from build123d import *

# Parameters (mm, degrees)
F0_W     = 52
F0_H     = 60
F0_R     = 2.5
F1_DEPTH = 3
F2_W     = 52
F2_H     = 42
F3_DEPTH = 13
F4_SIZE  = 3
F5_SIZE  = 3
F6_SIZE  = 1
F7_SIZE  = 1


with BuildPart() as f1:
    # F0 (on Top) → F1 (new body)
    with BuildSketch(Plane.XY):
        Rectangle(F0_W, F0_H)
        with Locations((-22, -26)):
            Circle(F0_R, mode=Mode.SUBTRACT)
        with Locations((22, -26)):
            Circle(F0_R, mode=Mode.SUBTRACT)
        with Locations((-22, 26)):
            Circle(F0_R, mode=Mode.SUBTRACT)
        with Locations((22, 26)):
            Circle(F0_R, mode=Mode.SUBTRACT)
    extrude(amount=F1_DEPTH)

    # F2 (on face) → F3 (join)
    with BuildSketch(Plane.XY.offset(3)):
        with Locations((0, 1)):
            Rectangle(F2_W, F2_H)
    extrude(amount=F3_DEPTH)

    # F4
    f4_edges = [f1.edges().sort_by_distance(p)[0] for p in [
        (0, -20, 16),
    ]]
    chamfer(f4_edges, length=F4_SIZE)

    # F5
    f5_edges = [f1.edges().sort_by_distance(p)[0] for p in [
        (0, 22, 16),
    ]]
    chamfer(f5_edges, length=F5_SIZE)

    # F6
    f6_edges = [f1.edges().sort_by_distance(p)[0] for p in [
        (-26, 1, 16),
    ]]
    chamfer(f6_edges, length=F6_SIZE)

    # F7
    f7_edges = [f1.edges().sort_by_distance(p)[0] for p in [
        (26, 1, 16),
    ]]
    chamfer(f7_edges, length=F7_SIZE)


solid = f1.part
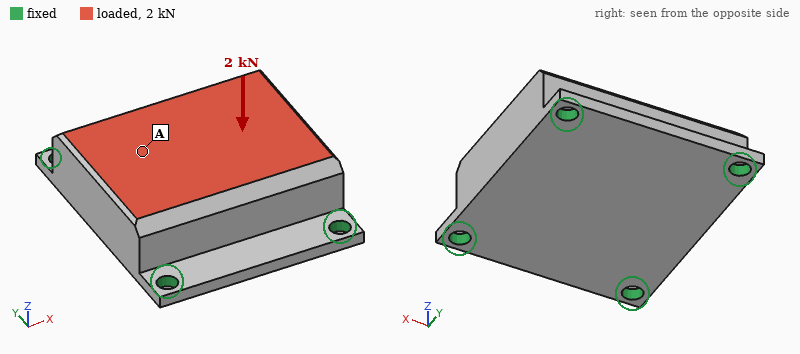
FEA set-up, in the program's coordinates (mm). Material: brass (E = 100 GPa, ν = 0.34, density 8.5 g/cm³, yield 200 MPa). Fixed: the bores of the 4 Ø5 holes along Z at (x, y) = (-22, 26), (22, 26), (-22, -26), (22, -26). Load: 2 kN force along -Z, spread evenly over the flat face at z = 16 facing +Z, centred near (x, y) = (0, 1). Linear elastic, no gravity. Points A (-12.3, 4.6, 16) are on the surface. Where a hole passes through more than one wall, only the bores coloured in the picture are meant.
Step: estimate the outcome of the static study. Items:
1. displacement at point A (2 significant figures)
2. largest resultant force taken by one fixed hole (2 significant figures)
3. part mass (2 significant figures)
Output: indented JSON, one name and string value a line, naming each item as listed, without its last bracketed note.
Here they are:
{
  "displacement at point A": "5.9 µm",
  "largest resultant force taken by one fixed hole": "620 N",
  "part mass": "310 g"
}
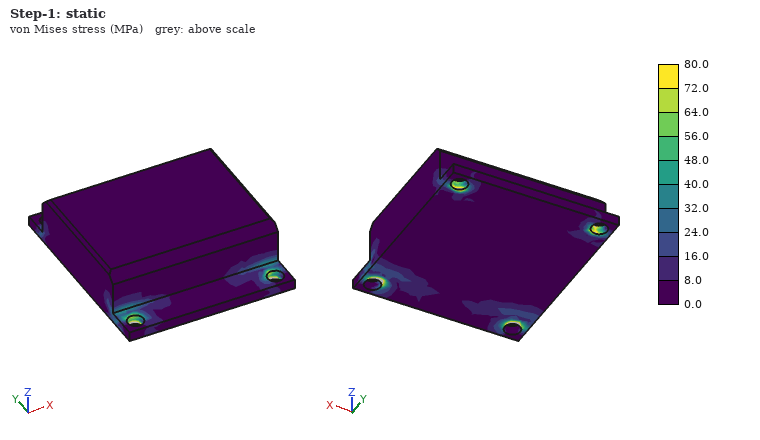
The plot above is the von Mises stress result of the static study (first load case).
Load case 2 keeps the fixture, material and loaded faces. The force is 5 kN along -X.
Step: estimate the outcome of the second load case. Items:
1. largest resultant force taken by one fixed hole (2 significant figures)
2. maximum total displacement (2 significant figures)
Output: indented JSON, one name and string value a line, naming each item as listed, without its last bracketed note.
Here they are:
{
  "largest resultant force taken by one fixed hole": "2.0 kN",
  "maximum total displacement": "16 µm"
}
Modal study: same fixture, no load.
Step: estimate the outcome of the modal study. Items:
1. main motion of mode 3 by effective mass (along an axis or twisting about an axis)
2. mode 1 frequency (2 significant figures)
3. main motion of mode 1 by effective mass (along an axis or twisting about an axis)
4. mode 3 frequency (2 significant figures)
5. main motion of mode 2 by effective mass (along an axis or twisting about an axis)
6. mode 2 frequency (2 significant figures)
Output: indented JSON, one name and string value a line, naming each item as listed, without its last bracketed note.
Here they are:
{
  "main motion of mode 3 by effective mass": "along Y",
  "mode 1 frequency": "5400 Hz",
  "main motion of mode 1 by effective mass": "along Z",
  "mode 3 frequency": "8900 Hz",
  "main motion of mode 2 by effective mass": "along X",
  "mode 2 frequency": "7000 Hz"
}
